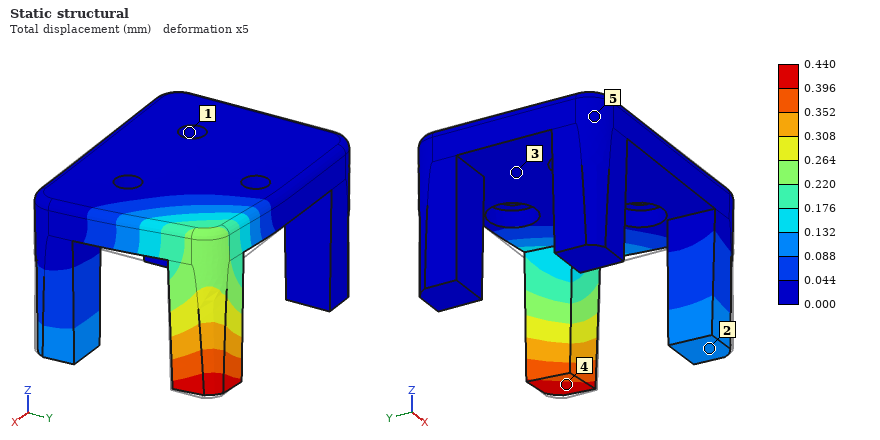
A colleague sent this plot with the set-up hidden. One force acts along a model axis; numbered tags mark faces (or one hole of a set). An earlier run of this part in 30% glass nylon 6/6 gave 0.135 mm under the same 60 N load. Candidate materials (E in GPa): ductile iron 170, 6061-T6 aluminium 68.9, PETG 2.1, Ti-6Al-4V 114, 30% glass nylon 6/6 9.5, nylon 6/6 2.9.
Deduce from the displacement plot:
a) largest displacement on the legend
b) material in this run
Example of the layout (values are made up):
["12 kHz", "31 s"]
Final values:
["0.440 mm", "nylon 6/6"]
